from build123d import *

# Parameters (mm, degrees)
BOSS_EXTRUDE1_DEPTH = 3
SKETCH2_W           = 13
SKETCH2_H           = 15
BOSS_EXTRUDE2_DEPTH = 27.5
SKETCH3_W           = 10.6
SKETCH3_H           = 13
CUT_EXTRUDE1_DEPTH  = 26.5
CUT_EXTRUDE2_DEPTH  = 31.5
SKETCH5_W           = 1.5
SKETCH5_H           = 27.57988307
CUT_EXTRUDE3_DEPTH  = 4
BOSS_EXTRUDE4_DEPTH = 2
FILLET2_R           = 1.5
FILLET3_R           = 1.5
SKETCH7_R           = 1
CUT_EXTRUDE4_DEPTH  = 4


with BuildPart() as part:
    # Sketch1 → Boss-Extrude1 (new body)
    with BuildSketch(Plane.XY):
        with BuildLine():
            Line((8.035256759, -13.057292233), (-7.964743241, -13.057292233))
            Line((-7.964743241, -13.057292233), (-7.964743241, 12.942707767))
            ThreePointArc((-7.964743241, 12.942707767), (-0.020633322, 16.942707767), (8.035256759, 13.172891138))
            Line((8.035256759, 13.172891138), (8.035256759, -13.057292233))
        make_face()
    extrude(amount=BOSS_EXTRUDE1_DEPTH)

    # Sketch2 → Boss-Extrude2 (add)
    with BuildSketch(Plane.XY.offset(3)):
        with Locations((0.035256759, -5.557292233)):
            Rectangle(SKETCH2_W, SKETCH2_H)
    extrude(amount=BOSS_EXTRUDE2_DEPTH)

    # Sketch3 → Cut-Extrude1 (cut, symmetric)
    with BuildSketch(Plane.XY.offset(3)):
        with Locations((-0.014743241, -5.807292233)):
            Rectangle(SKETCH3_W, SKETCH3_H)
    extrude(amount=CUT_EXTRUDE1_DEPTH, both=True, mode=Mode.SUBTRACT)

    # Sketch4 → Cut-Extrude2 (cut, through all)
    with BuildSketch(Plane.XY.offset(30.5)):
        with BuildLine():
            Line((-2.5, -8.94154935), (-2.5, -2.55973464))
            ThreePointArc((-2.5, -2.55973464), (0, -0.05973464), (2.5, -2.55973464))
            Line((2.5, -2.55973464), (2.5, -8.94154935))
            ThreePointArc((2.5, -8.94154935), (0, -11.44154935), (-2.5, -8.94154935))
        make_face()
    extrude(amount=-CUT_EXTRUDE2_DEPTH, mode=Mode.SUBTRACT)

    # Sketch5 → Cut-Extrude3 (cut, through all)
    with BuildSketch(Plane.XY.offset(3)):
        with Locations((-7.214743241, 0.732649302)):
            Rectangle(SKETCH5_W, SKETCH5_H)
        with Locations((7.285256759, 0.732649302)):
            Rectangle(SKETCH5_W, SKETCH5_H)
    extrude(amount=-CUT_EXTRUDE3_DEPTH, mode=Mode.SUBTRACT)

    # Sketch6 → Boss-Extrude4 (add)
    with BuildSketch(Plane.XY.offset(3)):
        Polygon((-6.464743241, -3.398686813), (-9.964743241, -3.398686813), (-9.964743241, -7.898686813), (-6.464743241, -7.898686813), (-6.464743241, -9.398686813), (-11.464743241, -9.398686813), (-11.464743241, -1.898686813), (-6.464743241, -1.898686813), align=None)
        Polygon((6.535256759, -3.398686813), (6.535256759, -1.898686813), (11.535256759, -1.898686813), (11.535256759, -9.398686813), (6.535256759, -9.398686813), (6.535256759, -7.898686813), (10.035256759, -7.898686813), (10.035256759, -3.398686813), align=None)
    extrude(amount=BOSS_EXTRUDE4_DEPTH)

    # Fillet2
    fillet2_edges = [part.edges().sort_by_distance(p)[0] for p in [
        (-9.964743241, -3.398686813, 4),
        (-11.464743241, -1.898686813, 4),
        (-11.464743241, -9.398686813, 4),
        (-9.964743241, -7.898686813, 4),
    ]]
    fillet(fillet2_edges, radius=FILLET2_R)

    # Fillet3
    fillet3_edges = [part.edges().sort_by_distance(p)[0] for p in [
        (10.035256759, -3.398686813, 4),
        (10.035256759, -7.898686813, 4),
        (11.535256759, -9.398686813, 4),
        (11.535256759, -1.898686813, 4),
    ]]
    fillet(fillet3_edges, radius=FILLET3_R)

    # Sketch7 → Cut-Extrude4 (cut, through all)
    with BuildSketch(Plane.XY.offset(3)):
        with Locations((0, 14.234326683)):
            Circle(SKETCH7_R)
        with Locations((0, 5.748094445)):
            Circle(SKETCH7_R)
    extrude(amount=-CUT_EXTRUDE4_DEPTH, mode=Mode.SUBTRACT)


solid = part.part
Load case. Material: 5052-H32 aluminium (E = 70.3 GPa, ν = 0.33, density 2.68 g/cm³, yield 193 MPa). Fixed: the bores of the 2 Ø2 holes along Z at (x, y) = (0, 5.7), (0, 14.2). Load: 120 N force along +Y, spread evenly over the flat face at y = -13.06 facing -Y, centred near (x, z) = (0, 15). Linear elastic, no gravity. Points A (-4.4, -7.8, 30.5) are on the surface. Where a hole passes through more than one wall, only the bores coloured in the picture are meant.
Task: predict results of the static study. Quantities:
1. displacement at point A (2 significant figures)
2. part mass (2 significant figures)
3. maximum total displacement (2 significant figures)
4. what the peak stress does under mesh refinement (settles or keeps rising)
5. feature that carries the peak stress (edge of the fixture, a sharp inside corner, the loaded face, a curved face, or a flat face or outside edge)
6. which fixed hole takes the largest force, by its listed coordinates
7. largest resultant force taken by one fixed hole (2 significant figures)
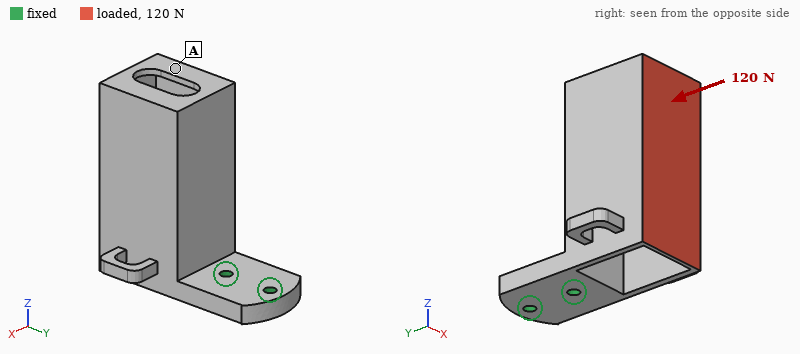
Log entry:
0.27 mm
6.6 g
0.29 mm
keeps rising
edge of the fixture
(0, 5.7)
120 N
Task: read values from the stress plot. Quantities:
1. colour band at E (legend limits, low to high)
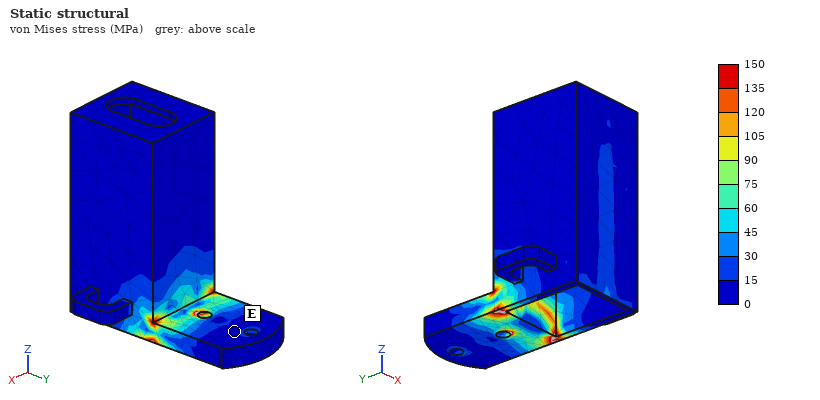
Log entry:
0 to 15 MPa
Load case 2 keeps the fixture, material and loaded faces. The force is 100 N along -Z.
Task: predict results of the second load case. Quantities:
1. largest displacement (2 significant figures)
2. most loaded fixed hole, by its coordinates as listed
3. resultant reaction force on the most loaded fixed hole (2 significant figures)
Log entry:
0.28 mm
(0, 5.7)
190 N
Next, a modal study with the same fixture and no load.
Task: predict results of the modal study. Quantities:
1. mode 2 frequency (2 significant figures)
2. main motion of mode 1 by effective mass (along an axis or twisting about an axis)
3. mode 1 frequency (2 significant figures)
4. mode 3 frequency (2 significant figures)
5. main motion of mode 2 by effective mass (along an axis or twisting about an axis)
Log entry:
2600 Hz
along Y
1600 Hz
4100 Hz
along X
